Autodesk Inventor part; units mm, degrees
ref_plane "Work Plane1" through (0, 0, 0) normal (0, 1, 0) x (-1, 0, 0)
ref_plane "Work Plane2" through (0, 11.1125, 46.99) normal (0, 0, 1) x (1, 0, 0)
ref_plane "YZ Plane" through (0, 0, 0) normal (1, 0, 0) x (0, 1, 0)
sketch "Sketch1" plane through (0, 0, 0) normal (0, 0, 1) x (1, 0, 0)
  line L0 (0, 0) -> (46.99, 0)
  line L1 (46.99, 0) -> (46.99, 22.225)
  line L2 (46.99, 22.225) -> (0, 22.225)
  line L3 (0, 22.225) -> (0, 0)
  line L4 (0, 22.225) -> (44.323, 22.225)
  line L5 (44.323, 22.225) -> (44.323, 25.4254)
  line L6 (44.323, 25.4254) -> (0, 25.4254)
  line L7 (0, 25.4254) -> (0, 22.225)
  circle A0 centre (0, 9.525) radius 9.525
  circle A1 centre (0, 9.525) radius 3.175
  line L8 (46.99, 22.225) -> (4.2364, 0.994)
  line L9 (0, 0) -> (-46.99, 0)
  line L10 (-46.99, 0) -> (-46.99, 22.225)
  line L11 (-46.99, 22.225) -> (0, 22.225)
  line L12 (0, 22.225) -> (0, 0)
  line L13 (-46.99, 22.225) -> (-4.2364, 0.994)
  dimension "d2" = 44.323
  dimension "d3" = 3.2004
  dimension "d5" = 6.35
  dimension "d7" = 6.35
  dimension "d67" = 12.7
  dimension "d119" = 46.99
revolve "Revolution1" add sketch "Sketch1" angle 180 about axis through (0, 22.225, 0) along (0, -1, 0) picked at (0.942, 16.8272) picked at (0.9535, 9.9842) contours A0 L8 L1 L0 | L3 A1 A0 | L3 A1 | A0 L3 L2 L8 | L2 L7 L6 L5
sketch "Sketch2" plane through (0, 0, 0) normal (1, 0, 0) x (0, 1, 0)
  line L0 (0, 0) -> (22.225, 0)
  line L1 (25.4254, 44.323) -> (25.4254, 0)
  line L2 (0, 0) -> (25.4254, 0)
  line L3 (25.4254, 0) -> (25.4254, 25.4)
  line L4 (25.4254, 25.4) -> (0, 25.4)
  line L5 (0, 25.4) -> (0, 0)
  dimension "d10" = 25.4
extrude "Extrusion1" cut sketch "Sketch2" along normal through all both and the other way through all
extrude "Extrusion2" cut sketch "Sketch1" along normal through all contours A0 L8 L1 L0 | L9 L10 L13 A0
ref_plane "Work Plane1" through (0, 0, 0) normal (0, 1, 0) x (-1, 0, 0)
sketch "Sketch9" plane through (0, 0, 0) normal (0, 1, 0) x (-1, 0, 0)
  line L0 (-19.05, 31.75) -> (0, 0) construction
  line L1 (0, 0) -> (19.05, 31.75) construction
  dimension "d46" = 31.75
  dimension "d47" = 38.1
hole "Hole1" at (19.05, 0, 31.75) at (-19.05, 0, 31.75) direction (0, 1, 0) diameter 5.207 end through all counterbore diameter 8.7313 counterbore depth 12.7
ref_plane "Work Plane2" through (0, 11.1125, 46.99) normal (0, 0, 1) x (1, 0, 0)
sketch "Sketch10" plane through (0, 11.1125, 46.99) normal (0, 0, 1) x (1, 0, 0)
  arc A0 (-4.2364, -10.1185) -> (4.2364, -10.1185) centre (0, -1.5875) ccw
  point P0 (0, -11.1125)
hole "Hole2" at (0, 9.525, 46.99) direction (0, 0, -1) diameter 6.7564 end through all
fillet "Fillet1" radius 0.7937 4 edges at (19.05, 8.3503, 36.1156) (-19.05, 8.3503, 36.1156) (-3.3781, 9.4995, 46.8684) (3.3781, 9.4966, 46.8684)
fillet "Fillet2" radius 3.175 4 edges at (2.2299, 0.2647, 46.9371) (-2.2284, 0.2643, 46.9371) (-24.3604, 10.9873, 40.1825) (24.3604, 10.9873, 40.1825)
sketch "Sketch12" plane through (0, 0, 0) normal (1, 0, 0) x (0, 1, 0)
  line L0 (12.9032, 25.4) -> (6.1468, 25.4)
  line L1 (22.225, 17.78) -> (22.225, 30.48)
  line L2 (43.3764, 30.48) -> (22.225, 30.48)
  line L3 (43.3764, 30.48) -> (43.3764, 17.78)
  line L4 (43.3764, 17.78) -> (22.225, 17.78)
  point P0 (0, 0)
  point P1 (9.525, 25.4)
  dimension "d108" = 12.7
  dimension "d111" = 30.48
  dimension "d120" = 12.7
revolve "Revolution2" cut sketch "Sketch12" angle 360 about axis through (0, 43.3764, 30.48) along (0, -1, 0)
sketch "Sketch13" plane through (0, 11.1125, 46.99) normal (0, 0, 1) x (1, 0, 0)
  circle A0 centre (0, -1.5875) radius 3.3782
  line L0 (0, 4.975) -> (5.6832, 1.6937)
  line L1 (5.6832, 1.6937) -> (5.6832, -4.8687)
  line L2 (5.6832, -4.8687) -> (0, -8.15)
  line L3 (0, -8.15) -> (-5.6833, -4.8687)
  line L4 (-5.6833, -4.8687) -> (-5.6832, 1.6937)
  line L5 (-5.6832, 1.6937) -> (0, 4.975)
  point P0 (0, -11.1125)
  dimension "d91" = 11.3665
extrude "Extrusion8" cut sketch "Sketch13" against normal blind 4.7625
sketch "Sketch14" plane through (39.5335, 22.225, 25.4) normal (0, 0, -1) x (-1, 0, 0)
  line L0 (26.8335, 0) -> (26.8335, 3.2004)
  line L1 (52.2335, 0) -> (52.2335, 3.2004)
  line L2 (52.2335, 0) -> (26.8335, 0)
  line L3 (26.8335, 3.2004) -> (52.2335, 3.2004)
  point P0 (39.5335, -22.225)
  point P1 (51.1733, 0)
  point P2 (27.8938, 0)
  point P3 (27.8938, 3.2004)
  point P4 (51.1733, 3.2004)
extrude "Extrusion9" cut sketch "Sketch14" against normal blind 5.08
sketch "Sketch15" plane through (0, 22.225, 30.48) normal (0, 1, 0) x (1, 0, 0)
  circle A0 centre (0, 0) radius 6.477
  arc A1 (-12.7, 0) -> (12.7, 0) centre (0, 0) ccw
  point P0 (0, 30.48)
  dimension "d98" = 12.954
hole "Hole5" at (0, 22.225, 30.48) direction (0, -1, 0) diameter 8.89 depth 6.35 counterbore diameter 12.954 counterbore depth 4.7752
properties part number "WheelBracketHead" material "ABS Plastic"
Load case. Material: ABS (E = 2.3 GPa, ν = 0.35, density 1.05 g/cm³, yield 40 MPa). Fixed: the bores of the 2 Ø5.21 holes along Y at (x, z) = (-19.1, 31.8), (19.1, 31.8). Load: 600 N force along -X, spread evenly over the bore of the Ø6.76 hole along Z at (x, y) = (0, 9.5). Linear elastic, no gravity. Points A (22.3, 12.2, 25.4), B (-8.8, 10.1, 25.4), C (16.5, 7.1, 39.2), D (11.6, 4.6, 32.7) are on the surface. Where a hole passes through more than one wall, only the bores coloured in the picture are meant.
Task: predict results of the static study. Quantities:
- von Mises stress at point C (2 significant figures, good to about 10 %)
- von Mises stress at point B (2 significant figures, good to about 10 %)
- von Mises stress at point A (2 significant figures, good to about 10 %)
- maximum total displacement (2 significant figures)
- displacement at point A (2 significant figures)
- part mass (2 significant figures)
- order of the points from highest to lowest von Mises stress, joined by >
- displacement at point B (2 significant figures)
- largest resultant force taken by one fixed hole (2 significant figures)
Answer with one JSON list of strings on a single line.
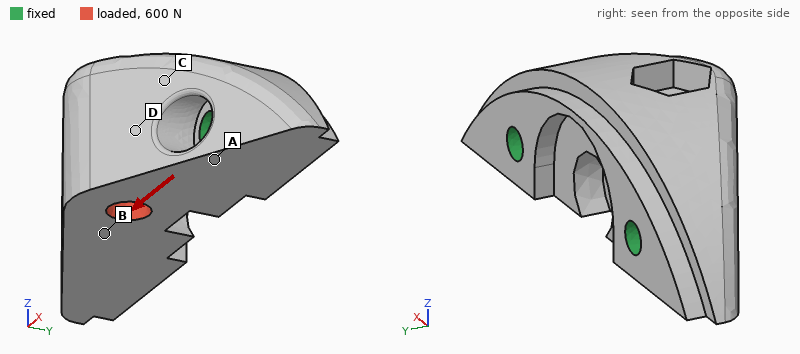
["1.1 MPa", "2.3 MPa", "1.7 MPa", "25 µm", "4.5 µm", "19 g", "B > A > C > D", "15 µm", "320 N"]
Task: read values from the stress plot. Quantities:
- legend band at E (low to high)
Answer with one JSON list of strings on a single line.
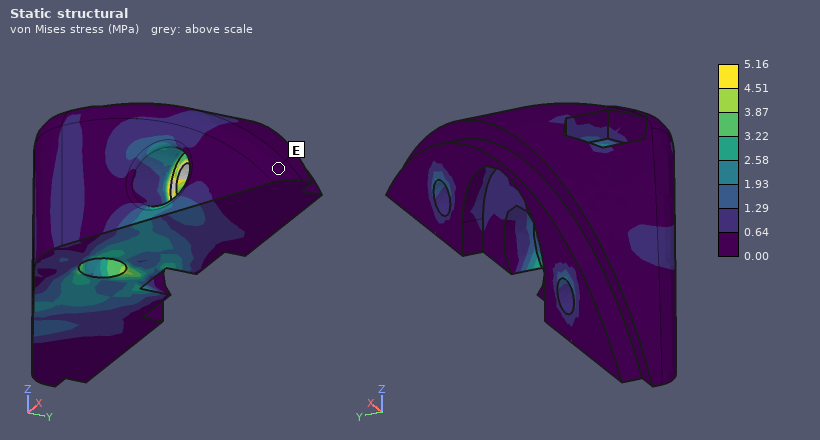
["0.00 to 0.64 MPa"]
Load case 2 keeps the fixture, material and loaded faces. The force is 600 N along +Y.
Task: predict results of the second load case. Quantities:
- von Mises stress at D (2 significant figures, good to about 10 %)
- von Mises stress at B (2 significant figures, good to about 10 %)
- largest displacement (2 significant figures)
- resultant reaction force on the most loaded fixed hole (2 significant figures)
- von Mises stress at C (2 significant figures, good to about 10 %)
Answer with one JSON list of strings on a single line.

["1.4 MPa", "2.2 MPa", "37 µm", "340 N", "0.93 MPa"]
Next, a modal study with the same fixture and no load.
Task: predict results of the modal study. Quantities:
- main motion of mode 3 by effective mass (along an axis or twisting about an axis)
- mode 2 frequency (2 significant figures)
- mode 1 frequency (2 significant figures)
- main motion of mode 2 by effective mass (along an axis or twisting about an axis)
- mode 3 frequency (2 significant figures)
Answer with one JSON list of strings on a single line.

["along X", "8100 Hz", "4800 Hz", "along Y", "9500 Hz"]
